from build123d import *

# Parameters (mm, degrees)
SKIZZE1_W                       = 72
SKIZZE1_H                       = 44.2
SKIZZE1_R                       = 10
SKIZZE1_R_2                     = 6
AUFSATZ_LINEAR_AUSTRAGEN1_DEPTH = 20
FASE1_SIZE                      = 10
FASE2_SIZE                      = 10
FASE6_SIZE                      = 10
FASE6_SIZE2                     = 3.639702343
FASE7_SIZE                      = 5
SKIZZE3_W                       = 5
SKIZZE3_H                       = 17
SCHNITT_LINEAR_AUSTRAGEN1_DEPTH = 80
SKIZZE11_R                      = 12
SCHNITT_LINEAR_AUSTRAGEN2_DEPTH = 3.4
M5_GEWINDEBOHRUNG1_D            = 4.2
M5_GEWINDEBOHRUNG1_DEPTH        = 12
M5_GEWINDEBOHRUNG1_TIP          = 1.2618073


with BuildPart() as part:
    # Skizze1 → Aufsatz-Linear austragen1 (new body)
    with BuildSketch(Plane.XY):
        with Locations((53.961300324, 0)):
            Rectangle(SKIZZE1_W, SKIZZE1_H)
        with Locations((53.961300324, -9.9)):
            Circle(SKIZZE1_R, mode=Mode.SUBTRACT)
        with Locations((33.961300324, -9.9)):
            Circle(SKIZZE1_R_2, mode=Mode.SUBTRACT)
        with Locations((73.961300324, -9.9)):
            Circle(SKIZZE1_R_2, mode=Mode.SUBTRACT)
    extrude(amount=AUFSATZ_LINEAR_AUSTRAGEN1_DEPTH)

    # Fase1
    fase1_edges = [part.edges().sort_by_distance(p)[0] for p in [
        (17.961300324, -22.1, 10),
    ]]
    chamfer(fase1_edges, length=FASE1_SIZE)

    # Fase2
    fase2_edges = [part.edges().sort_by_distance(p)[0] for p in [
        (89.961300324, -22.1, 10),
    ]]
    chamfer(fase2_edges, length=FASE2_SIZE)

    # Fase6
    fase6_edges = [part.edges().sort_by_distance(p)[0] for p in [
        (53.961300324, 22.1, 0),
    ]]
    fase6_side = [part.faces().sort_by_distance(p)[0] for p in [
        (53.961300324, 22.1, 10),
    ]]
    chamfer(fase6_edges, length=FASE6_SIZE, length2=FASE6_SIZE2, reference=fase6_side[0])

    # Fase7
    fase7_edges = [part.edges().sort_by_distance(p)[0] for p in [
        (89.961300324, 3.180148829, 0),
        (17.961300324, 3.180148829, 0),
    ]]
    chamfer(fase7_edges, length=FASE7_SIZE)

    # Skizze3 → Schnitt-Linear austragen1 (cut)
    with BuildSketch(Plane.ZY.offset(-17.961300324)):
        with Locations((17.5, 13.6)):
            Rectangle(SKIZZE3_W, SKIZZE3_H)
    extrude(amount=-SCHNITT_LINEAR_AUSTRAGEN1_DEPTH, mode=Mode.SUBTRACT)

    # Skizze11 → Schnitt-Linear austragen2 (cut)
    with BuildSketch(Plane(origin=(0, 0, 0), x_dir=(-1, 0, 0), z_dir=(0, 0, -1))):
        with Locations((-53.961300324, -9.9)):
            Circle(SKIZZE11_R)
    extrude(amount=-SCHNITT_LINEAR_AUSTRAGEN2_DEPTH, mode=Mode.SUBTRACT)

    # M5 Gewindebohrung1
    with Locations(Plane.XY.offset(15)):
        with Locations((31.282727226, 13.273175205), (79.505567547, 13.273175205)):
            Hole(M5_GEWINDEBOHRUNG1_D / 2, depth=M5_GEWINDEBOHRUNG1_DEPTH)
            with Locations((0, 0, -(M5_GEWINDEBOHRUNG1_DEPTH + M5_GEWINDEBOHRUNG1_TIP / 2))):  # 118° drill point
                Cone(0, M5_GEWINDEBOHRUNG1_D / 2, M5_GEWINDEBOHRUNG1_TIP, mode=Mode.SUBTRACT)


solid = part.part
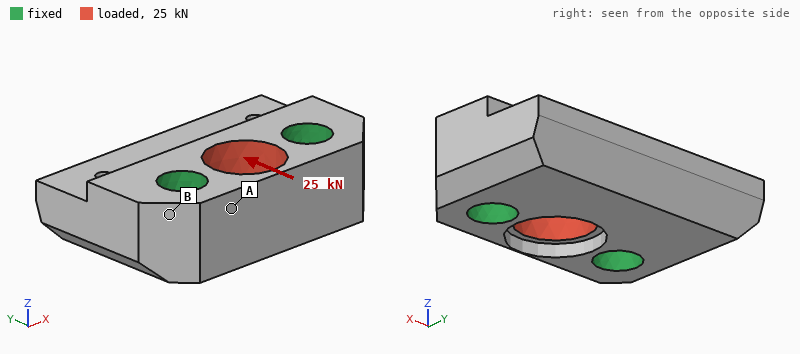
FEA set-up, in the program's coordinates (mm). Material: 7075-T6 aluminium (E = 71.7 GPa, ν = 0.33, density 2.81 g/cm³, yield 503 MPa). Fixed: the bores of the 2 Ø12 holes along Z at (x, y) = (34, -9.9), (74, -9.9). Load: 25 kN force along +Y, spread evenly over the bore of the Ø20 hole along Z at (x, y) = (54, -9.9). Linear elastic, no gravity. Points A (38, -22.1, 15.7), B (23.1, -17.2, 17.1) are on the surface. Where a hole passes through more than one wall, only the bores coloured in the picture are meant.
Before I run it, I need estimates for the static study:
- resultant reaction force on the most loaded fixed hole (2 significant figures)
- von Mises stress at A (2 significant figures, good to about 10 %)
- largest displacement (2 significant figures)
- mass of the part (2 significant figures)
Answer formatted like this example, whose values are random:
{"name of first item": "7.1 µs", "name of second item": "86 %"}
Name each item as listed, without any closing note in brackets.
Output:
{"resultant reaction force on the most loaded fixed hole": "13 kN", "von Mises stress at A": "39 MPa", "largest displacement": "44 µm", "mass of the part": "120 g"}
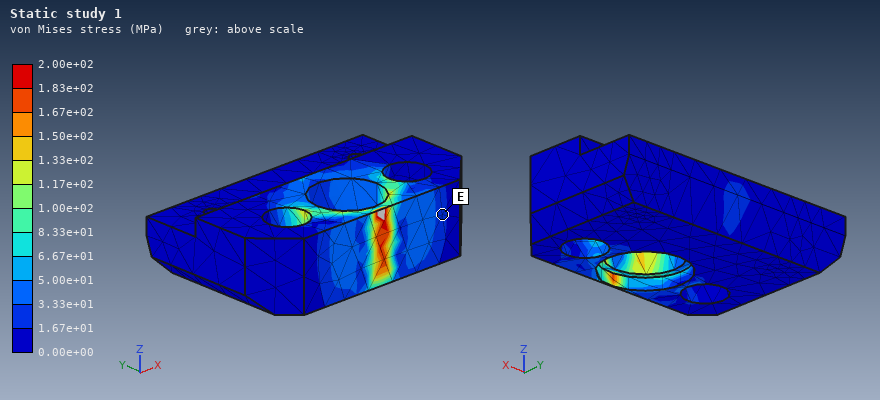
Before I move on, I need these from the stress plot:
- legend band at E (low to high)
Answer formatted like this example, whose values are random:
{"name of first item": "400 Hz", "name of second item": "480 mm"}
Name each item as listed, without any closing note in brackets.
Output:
{"legend band at E": "1.67e+01 to 3.33e+01 MPa"}
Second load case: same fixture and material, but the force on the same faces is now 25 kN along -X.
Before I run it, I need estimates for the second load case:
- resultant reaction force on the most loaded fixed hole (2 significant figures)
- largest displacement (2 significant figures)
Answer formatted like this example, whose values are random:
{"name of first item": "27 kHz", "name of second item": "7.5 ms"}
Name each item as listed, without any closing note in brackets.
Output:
{"resultant reaction force on the most loaded fixed hole": "13 kN", "largest displacement": "11 µm"}
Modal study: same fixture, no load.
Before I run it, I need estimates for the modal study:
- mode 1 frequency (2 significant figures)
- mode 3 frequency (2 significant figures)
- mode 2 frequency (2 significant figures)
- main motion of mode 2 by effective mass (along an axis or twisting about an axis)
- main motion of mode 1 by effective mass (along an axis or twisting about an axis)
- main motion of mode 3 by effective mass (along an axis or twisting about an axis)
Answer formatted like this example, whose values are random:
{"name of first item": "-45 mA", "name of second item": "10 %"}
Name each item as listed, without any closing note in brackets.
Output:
{"mode 1 frequency": "15 kHz", "mode 3 frequency": "21 kHz", "mode 2 frequency": "19 kHz", "main motion of mode 2 by effective mass": "twisting about Y", "main motion of mode 1 by effective mass": "along Z", "main motion of mode 3 by effective mass": "along X"}
